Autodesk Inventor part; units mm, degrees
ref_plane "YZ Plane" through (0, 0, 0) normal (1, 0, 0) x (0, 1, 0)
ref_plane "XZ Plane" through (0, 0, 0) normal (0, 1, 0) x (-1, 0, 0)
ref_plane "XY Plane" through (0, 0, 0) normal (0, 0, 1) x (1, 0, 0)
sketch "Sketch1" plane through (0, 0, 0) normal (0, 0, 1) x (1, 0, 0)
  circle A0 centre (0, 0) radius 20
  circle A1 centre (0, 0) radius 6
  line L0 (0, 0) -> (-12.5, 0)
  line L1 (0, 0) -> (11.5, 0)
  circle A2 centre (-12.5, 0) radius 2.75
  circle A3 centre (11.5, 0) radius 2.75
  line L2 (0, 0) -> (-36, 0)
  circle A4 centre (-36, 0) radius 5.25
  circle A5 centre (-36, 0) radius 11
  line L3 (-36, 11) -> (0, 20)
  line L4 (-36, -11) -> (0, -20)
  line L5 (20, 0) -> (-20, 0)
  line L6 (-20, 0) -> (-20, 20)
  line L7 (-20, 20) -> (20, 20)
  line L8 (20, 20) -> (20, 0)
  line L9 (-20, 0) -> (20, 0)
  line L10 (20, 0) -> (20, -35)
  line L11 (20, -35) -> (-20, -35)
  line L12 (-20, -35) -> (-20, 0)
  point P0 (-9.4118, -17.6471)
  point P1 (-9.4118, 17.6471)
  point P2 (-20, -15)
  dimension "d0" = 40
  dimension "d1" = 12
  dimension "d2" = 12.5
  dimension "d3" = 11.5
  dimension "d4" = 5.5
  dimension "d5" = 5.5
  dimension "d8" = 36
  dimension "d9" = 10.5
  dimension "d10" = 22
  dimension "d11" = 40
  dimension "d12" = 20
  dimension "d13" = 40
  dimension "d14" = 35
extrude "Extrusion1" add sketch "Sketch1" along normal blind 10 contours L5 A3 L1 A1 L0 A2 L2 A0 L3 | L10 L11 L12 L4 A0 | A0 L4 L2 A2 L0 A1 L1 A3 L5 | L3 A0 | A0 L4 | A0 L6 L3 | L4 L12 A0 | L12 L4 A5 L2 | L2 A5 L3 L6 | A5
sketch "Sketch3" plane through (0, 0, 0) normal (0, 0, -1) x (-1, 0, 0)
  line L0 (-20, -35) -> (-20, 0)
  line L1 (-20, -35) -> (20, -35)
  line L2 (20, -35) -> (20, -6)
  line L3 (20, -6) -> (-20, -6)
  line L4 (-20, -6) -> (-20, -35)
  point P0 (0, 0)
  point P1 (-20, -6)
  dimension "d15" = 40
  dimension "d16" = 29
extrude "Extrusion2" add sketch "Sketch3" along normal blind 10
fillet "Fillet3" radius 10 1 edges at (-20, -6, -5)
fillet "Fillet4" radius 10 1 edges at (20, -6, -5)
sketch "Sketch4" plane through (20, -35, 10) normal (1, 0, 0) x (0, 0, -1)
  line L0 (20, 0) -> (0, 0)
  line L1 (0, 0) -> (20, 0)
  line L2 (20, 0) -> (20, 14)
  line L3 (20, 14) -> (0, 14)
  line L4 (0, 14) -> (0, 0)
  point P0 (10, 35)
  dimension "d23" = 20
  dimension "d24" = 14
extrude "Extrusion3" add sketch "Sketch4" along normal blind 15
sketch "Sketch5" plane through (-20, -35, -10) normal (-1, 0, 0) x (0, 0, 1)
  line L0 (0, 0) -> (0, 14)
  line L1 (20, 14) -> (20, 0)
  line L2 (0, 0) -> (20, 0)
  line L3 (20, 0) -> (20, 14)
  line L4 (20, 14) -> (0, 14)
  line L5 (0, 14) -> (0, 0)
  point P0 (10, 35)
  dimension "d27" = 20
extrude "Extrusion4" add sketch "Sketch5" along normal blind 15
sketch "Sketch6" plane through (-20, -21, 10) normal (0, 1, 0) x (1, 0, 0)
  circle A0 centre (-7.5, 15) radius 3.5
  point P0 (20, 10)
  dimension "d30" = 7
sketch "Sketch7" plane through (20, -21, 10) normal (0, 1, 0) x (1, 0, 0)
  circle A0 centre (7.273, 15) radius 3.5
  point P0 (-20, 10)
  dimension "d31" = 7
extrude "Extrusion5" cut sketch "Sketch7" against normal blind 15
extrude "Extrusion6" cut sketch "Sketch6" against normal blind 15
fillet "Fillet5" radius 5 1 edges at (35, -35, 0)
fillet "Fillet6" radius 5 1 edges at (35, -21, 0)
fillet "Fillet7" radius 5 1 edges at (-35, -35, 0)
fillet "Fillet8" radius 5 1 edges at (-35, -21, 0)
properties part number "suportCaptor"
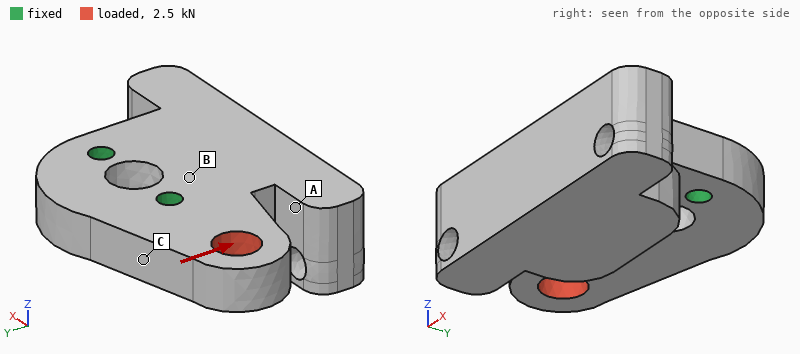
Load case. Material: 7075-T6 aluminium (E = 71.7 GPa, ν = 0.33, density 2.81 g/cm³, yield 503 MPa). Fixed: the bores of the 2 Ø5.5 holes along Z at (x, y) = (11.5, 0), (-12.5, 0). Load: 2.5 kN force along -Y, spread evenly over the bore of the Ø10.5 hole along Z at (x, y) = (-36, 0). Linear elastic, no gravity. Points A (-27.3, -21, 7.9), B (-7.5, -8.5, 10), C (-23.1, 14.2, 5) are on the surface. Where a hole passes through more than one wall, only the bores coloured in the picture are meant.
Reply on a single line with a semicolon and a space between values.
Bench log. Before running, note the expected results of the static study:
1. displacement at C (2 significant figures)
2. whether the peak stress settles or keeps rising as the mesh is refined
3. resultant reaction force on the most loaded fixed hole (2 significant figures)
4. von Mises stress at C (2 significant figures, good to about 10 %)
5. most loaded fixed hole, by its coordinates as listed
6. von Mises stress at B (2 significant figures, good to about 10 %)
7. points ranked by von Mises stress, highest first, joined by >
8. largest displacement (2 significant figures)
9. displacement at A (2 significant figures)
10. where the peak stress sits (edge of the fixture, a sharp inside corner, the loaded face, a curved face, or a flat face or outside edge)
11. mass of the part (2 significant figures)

14 µm; keeps rising; 4.1 kN; 31 MPa; (-12.5, 0); 18 MPa; C > B > A; 40 µm; 8.4 µm; edge of the fixture; 120 g
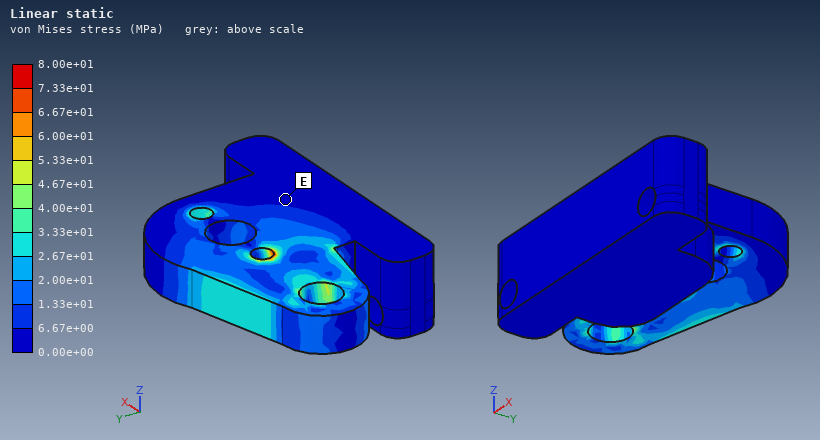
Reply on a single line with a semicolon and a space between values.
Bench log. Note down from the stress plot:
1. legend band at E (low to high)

0.00e+00 to 6.67e+00 MPa
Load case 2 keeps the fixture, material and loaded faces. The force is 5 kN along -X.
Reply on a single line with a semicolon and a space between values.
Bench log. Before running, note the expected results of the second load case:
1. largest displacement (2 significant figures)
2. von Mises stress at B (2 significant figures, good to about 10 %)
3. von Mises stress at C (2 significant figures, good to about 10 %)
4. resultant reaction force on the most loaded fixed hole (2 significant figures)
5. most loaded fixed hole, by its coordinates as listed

14 µm; 7.6 MPa; 13 MPa; 4.1 kN; (-12.5, 0)
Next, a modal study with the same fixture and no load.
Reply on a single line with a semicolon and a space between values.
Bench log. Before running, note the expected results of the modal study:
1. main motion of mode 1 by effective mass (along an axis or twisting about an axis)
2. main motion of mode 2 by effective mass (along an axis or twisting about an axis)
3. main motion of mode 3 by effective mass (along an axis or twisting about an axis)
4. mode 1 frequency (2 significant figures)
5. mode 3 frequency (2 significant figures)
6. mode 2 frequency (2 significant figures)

along Z; twisting about Y; along X; 3700 Hz; 8400 Hz; 7200 Hz
